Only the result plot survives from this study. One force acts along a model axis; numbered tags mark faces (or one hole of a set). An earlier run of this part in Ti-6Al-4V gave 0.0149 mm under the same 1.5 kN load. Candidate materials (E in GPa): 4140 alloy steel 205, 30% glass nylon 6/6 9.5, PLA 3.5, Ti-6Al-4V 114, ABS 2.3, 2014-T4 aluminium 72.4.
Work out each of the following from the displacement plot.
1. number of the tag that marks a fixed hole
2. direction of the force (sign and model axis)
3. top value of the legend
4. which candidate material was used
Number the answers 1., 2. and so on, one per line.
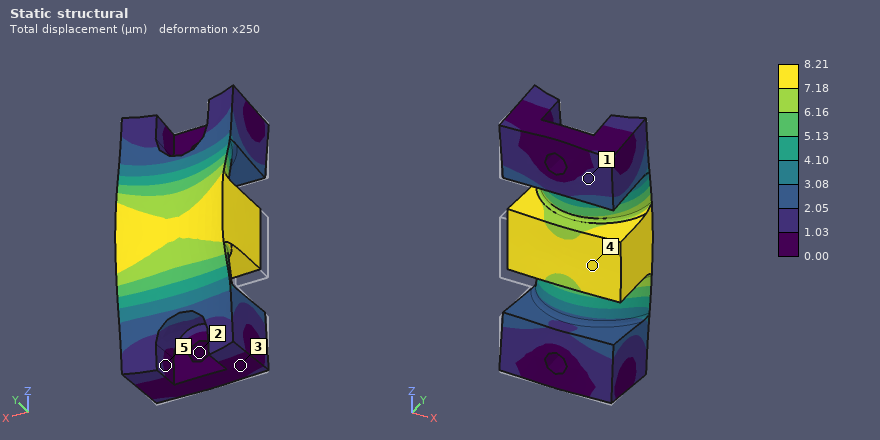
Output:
1. 2
2. +Y
3. 8.21 µm
4. 4140 alloy steel
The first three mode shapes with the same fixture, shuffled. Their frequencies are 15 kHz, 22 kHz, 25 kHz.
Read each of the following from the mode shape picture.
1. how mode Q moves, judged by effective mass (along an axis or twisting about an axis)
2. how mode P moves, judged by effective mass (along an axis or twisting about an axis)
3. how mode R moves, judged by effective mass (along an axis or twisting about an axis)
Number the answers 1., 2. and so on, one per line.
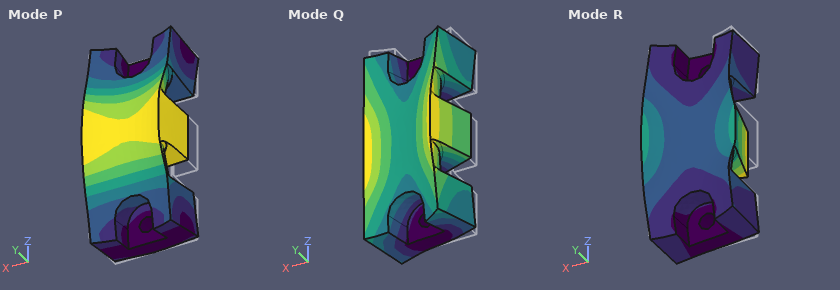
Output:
1. along X
2. along Y
3. along X
